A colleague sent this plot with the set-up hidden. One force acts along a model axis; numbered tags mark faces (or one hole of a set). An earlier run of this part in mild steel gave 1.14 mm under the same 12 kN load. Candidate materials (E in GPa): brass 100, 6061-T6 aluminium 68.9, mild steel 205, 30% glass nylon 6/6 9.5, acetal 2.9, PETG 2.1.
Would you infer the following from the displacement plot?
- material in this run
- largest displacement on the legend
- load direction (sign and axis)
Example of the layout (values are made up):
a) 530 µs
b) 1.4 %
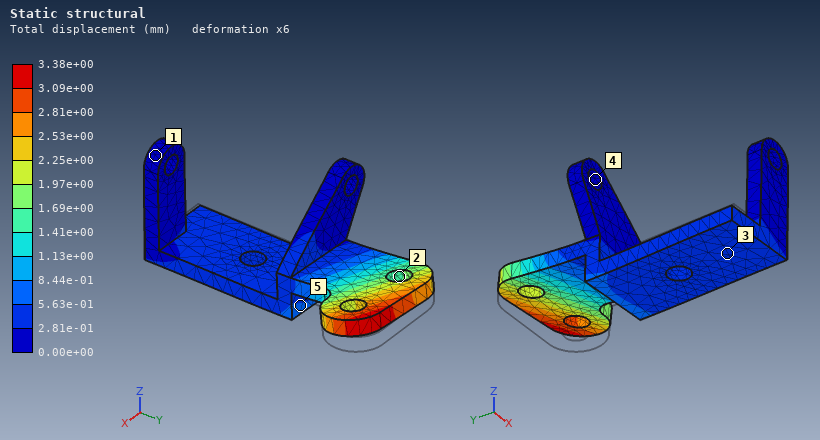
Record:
a) 6061-T6 aluminium
b) 3.38e+00 mm
c) +Z
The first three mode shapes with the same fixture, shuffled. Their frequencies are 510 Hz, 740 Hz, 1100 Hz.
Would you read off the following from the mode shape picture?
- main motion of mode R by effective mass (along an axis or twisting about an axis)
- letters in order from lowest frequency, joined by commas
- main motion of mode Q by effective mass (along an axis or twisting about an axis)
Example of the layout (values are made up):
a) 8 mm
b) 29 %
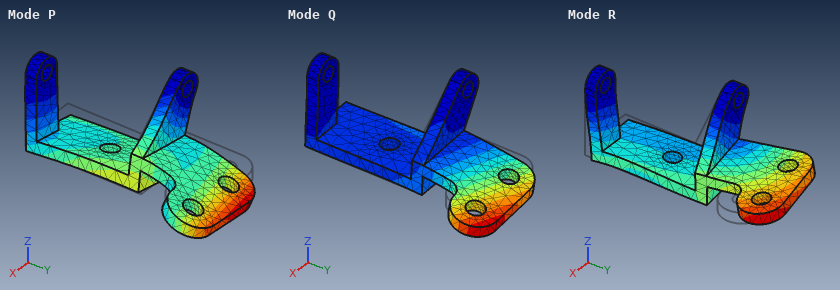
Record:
a) along Y
b) Q, R, P
c) along Z
